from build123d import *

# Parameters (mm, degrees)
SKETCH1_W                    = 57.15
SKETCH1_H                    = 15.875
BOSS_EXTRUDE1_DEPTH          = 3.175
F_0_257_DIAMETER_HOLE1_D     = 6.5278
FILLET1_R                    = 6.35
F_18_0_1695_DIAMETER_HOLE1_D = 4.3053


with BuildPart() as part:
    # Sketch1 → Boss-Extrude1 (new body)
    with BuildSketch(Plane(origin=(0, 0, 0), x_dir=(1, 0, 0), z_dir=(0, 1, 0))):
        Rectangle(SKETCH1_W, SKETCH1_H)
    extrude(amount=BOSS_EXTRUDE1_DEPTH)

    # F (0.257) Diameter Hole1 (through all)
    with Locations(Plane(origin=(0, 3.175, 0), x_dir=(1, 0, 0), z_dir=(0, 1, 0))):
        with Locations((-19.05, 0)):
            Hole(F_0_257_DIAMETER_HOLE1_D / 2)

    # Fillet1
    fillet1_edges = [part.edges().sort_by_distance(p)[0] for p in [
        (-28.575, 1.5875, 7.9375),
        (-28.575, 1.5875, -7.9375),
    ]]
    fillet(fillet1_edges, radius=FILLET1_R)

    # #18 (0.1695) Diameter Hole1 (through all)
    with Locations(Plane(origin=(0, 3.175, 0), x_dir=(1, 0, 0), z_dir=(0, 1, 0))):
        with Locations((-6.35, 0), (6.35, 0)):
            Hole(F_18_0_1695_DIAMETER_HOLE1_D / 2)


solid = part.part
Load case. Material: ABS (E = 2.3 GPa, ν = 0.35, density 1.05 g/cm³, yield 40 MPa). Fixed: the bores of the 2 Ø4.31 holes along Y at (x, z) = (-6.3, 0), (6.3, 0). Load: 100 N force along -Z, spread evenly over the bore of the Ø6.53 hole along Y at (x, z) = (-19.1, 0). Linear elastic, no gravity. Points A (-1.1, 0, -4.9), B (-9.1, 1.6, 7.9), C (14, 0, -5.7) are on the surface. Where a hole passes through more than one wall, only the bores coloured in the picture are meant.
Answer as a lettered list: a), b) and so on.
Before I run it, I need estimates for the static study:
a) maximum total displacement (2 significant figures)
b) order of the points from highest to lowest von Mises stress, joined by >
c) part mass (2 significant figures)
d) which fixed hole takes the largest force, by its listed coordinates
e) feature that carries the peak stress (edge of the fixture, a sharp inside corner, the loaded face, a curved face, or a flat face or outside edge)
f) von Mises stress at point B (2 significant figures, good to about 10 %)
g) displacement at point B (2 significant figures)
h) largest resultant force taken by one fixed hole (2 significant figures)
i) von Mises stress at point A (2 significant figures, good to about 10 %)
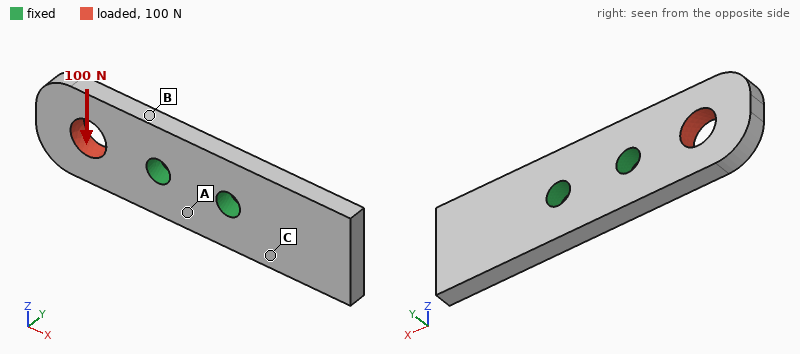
a) 0.17 mm
b) B > A > C
c) 2.8 g
d) (-6.3, 0)
e) edge of the fixture
f) 8.2 MPa
g) 0.038 mm
h) 150 N
i) 3.1 MPa
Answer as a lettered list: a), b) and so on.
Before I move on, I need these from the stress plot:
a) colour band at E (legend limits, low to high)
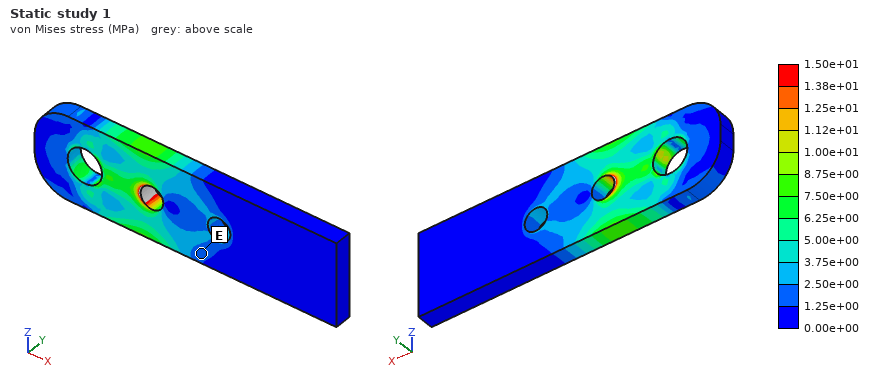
a) 1.25e+00 to 2.50e+00 MPa
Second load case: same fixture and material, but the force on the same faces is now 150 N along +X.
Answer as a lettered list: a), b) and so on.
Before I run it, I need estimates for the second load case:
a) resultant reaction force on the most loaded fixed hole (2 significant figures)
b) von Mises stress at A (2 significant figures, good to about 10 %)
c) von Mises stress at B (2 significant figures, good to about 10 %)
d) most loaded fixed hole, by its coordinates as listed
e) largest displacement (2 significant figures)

a) 130 N
b) 1.0 MPa
c) 2.1 MPa
d) (-6.3, 0)
e) 33 µm
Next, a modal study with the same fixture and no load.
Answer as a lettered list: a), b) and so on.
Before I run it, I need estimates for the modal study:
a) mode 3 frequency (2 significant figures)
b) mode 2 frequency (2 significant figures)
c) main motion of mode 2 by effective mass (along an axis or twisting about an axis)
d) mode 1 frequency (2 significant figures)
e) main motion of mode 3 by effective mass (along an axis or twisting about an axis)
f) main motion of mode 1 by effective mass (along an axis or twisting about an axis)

a) 4100 Hz
b) 1800 Hz
c) along Y
d) 1700 Hz
e) twisting about X
f) along Y
